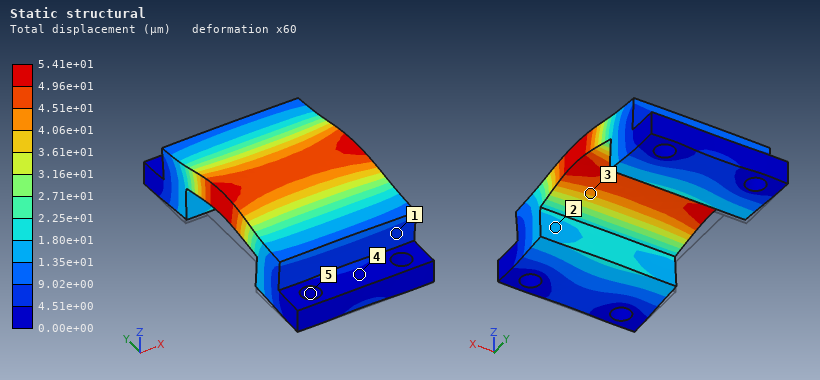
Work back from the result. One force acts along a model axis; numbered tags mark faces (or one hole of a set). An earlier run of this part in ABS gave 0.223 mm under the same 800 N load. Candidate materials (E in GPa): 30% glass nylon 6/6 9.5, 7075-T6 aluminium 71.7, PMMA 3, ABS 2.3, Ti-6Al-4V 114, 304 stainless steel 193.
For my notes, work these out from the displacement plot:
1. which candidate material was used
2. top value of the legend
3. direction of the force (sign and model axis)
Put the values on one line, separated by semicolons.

30% glass nylon 6/6; 5.41e+01 µm; +Z
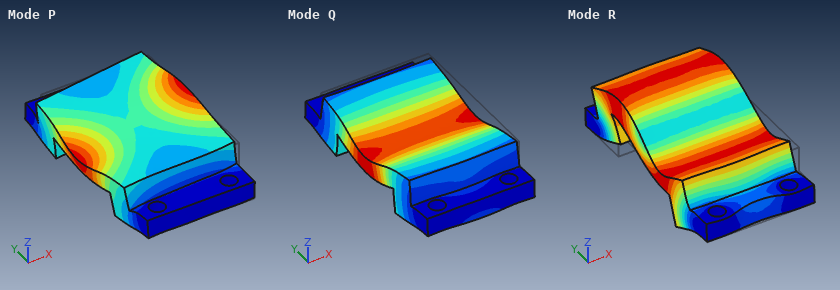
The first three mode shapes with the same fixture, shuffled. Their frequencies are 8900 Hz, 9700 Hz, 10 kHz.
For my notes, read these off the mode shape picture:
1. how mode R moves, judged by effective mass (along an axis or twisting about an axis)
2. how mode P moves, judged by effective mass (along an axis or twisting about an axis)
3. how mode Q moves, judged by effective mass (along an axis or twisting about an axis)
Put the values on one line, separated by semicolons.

along Y; along X; along Z
